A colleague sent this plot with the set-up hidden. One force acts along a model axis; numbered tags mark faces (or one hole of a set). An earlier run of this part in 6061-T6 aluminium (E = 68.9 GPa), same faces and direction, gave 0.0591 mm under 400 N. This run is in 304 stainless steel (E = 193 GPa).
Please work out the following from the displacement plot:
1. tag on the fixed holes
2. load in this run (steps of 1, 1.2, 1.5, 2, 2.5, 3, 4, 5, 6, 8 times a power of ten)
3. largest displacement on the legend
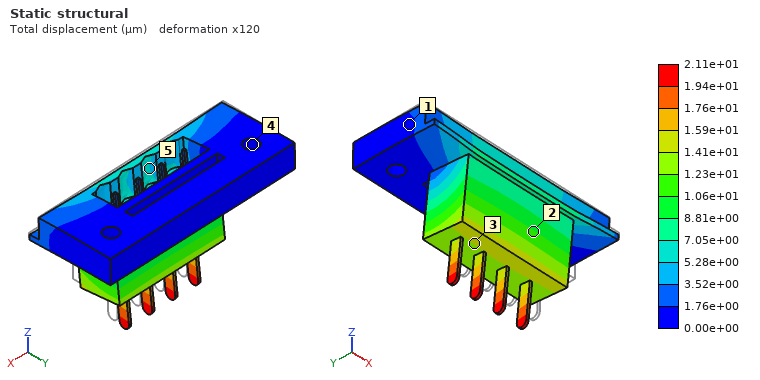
4
400 N
2.11e+01 µm
